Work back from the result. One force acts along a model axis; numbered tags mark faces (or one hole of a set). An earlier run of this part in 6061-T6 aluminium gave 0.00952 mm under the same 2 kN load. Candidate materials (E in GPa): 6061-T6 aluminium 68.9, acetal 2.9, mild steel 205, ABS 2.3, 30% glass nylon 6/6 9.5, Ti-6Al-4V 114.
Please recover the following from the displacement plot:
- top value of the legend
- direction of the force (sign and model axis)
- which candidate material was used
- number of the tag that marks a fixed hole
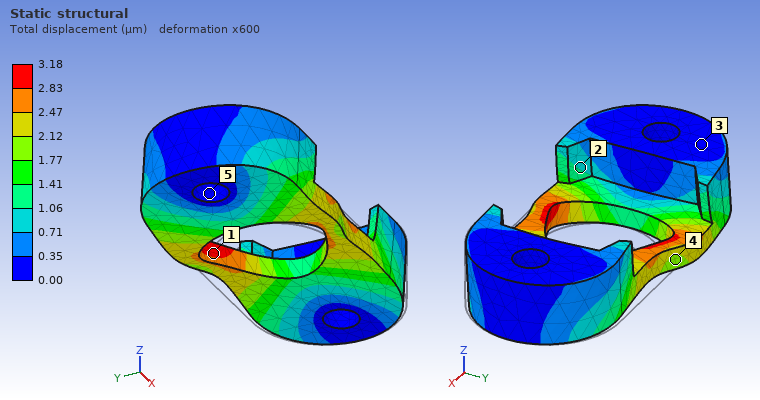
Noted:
3.18 µm
-X
mild steel
5
